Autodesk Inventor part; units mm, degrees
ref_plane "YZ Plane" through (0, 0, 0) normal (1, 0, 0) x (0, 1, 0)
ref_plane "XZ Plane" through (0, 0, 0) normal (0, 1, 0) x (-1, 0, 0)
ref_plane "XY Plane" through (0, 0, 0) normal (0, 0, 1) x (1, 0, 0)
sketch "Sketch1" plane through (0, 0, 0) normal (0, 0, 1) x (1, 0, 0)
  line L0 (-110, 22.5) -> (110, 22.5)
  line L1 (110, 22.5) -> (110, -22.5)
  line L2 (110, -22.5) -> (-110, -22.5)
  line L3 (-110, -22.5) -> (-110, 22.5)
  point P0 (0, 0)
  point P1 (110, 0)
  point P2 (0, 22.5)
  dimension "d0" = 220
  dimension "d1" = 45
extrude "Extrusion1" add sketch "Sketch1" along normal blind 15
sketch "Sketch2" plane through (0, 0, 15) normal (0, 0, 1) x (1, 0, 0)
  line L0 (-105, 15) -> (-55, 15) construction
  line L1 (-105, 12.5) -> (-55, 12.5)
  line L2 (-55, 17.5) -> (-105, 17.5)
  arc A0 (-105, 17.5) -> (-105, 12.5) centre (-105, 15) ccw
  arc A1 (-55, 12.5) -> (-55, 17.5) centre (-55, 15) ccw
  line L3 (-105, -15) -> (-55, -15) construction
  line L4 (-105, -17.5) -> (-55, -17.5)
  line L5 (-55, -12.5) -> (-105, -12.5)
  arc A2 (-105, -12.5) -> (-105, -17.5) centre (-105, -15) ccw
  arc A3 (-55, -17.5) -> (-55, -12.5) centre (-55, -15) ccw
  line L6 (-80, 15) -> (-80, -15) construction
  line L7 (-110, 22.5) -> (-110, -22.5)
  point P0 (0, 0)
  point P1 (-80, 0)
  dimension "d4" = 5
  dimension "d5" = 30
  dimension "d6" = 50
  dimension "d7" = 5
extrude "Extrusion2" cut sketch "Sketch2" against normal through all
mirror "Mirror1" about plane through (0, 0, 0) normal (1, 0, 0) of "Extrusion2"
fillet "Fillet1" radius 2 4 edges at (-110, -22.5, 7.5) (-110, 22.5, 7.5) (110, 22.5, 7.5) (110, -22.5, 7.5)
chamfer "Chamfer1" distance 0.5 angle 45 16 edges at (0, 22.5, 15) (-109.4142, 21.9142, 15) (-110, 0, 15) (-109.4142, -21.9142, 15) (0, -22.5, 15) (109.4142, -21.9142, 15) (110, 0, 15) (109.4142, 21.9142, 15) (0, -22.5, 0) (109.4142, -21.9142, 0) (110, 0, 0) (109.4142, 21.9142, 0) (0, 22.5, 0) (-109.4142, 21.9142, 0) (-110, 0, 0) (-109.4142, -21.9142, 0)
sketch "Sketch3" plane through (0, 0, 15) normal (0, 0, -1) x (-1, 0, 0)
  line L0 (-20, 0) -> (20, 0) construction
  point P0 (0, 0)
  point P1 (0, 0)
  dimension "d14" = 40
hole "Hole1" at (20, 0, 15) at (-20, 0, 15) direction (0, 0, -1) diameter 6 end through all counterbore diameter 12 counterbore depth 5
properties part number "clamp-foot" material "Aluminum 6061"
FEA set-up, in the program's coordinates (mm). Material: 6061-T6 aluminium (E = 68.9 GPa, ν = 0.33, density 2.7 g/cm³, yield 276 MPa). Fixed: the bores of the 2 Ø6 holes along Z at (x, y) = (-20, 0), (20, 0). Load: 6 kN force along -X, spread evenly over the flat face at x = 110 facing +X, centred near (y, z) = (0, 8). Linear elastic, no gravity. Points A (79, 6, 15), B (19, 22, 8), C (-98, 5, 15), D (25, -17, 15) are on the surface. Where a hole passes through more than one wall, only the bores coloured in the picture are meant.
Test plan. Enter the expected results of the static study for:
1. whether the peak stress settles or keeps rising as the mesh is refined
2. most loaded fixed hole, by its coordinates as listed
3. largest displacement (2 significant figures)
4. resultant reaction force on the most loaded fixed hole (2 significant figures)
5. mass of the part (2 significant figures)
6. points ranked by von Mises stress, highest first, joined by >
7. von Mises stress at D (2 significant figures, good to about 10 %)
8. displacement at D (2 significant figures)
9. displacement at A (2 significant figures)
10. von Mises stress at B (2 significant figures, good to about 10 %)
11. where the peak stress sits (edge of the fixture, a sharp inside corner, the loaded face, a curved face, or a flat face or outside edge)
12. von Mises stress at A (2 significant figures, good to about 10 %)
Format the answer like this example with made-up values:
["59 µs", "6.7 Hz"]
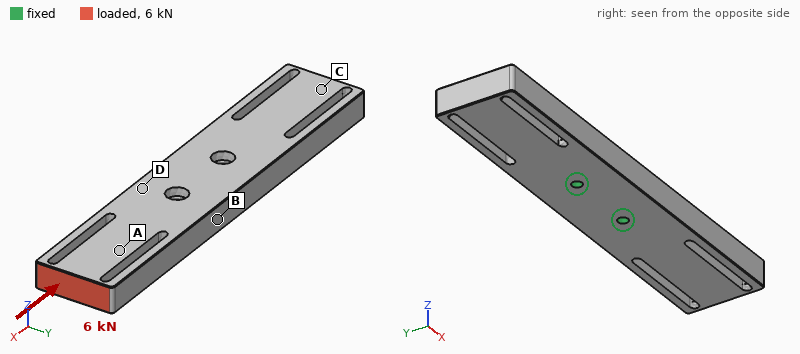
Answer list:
["keeps rising", "(20, 0)", "25 µm", "4.4 kN", "350 g", "A > D > B > C", "8.6 MPa", "4.5 µm", "16 µm", "5.7 MPa", "edge of the fixture", "12 MPa"]
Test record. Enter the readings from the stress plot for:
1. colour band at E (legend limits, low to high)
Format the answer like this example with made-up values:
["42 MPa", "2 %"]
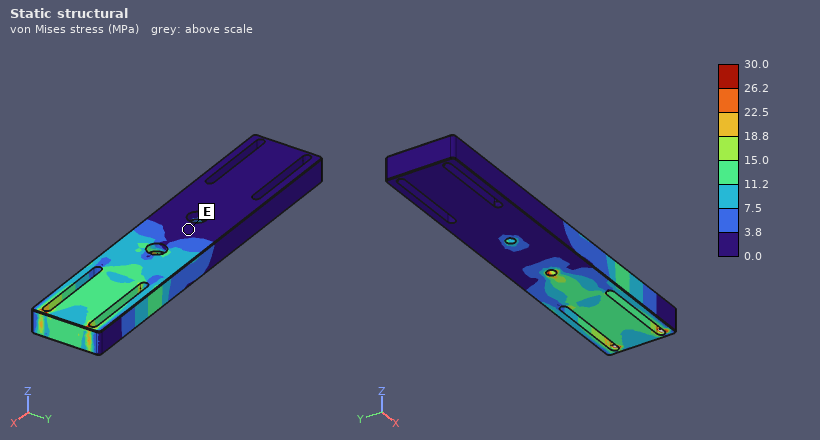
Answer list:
["0.0 to 3.8 MPa"]
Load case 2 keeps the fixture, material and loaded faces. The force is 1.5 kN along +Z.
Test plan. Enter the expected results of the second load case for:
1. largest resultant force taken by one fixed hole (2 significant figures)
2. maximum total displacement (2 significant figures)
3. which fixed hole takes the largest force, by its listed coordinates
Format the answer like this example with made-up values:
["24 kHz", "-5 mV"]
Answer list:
["4.3 kN", "0.59 mm", "(20, 0)"]
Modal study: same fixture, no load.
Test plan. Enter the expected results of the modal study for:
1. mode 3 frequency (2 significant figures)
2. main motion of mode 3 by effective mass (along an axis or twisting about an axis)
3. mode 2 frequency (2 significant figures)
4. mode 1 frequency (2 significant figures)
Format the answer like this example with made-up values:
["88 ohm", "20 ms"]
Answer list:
["2500 Hz", "twisting about Z", "1400 Hz", "1400 Hz"]
